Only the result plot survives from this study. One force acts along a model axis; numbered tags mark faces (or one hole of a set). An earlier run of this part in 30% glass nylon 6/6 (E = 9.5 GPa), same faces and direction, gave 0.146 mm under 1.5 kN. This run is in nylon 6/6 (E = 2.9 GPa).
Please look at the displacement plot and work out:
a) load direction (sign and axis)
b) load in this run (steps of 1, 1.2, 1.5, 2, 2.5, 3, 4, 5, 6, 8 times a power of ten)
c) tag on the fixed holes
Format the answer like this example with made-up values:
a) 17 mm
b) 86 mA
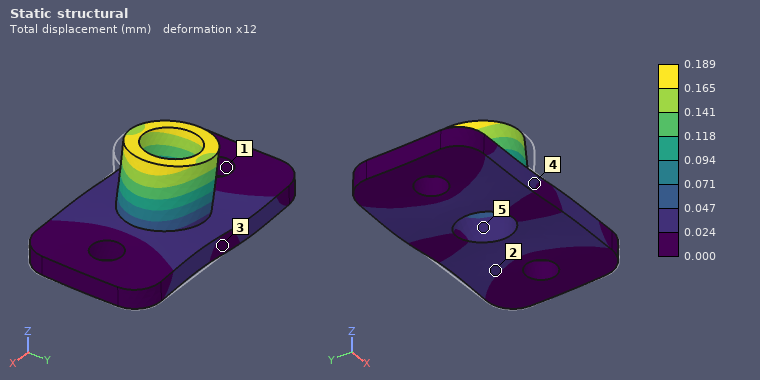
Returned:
a) -X
b) 600 N
c) 1
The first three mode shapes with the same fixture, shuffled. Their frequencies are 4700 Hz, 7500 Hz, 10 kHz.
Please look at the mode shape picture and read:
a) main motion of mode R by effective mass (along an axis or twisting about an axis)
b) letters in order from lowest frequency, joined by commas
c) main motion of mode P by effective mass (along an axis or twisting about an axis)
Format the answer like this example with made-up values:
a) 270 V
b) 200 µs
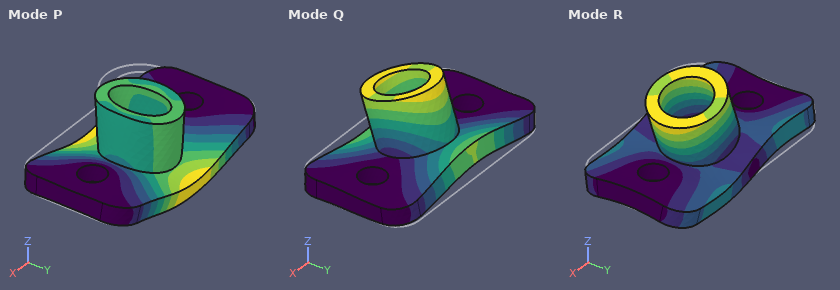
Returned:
a) along X
b) Q, P, R
c) along Z
